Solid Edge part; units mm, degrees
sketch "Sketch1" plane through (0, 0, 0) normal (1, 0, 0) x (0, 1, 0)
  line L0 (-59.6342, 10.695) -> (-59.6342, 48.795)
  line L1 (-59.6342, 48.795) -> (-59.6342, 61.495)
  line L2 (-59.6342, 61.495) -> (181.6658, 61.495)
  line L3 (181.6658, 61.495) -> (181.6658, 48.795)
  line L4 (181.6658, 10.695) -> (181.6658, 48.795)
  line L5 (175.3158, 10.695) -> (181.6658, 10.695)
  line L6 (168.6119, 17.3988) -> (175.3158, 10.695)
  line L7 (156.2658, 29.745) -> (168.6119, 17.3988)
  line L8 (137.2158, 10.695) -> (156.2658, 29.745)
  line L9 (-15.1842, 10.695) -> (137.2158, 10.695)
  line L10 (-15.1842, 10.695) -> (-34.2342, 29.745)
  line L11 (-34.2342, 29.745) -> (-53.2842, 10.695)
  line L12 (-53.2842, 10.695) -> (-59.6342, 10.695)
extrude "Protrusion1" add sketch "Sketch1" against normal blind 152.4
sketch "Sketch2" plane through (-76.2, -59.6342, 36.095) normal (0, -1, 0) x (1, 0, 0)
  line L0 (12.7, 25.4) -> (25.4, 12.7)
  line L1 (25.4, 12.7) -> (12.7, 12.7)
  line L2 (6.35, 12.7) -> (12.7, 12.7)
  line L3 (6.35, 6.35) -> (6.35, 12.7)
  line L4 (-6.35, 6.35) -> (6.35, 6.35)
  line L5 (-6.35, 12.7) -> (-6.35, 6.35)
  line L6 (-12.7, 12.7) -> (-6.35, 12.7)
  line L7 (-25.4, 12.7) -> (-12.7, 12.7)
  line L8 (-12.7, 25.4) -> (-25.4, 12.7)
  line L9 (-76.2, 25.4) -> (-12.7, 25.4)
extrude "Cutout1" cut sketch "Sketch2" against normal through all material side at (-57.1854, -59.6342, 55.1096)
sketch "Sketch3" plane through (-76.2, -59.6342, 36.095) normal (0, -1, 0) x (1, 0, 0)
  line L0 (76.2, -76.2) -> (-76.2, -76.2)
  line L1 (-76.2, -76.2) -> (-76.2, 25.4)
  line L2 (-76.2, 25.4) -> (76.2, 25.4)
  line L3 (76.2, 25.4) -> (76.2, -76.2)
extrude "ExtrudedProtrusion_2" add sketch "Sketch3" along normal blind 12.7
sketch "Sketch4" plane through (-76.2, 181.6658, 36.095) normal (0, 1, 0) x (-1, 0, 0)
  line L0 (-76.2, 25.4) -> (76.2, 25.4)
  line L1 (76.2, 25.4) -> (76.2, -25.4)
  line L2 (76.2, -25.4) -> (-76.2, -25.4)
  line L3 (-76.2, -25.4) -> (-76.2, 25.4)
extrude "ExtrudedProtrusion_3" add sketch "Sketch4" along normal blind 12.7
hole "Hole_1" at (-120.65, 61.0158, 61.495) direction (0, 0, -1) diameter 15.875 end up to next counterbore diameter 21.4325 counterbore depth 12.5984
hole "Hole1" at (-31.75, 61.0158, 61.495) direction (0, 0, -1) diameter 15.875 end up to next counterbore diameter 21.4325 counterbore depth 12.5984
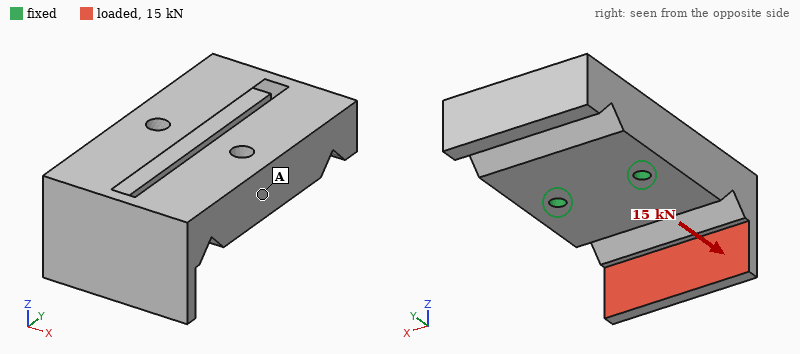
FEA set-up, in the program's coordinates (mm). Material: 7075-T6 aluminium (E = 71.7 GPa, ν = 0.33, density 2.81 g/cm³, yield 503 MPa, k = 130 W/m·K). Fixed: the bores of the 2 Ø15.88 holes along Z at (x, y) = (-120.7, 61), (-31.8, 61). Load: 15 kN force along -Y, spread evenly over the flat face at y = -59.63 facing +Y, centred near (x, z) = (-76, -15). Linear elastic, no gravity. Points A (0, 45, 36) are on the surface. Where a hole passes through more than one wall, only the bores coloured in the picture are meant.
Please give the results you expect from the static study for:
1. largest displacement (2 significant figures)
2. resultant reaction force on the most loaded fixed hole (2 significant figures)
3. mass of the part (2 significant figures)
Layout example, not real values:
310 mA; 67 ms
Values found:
0.37 mm; 7.7 kN; 5.3 kg
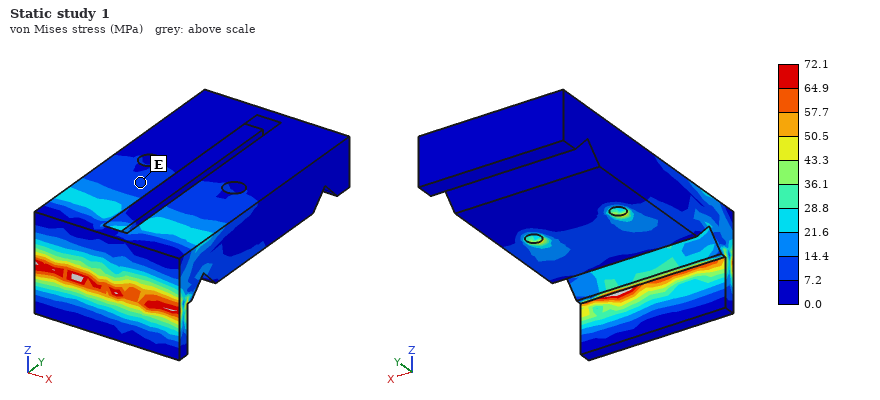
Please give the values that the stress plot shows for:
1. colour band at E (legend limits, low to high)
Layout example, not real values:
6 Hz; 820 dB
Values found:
7.2 to 14.4 MPa
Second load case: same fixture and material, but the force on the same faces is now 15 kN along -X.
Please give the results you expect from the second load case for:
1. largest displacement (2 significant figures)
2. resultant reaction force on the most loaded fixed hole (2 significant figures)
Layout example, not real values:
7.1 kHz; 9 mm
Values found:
0.16 mm; 21 kN
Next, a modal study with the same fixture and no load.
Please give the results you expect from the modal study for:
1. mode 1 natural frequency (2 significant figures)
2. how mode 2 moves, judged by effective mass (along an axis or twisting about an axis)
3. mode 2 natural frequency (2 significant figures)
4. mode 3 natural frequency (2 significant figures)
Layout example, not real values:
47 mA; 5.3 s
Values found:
1300 Hz; along Z; 1900 Hz; 2300 Hz
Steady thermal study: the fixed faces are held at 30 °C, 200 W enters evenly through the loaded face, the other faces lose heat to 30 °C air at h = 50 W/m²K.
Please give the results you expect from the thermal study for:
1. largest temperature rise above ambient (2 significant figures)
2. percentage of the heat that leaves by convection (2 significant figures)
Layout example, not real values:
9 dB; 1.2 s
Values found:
49 K; 36 %
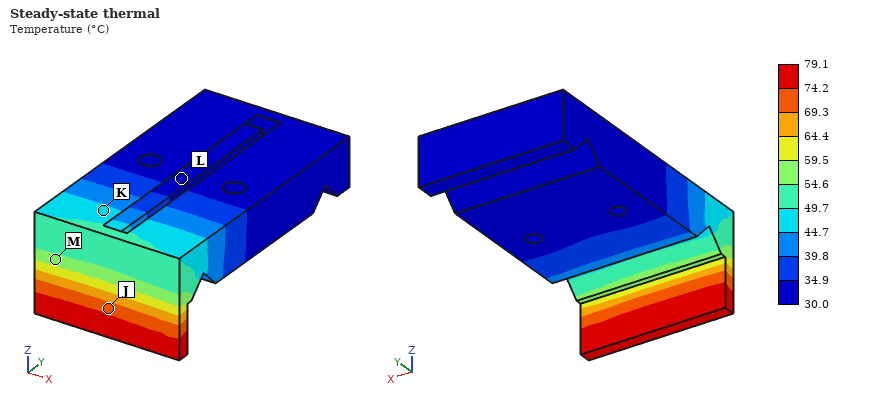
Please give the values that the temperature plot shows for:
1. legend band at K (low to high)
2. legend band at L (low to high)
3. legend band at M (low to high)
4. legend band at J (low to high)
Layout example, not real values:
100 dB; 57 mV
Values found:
44.7 to 49.7 °C; 30.0 to 34.9 °C; 54.6 to 59.5 °C; 69.3 to 74.2 °C
